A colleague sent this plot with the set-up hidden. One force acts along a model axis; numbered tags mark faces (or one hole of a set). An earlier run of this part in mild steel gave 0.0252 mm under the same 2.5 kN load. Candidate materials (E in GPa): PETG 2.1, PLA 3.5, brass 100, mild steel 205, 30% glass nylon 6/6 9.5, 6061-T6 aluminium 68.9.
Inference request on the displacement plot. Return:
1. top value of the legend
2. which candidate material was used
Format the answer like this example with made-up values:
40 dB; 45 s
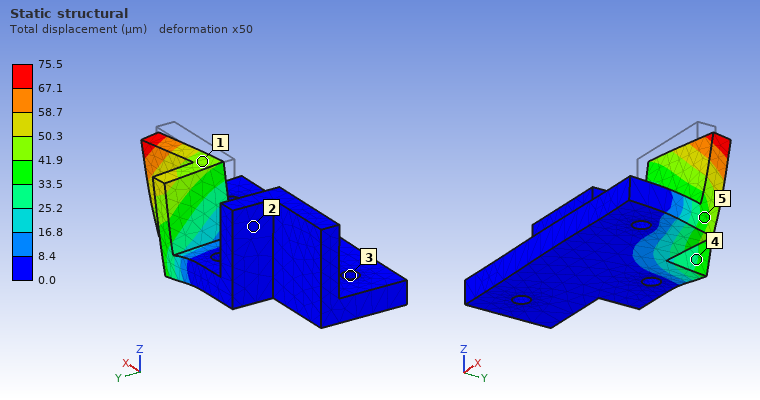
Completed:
75.5 µm; 6061-T6 aluminium
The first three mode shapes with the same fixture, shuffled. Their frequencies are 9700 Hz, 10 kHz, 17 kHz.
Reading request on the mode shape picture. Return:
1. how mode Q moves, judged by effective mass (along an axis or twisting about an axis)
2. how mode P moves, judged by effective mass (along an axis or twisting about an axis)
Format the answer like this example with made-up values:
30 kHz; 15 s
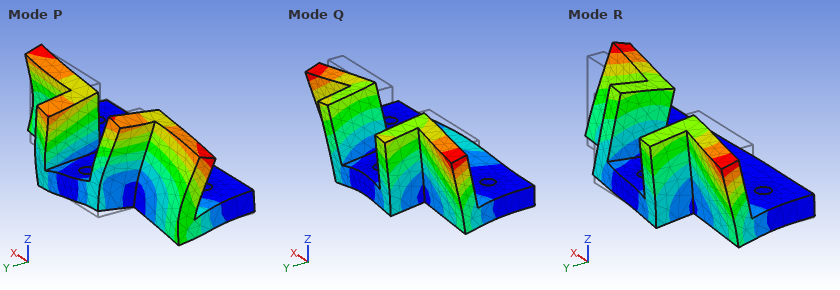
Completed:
along Y; along X
